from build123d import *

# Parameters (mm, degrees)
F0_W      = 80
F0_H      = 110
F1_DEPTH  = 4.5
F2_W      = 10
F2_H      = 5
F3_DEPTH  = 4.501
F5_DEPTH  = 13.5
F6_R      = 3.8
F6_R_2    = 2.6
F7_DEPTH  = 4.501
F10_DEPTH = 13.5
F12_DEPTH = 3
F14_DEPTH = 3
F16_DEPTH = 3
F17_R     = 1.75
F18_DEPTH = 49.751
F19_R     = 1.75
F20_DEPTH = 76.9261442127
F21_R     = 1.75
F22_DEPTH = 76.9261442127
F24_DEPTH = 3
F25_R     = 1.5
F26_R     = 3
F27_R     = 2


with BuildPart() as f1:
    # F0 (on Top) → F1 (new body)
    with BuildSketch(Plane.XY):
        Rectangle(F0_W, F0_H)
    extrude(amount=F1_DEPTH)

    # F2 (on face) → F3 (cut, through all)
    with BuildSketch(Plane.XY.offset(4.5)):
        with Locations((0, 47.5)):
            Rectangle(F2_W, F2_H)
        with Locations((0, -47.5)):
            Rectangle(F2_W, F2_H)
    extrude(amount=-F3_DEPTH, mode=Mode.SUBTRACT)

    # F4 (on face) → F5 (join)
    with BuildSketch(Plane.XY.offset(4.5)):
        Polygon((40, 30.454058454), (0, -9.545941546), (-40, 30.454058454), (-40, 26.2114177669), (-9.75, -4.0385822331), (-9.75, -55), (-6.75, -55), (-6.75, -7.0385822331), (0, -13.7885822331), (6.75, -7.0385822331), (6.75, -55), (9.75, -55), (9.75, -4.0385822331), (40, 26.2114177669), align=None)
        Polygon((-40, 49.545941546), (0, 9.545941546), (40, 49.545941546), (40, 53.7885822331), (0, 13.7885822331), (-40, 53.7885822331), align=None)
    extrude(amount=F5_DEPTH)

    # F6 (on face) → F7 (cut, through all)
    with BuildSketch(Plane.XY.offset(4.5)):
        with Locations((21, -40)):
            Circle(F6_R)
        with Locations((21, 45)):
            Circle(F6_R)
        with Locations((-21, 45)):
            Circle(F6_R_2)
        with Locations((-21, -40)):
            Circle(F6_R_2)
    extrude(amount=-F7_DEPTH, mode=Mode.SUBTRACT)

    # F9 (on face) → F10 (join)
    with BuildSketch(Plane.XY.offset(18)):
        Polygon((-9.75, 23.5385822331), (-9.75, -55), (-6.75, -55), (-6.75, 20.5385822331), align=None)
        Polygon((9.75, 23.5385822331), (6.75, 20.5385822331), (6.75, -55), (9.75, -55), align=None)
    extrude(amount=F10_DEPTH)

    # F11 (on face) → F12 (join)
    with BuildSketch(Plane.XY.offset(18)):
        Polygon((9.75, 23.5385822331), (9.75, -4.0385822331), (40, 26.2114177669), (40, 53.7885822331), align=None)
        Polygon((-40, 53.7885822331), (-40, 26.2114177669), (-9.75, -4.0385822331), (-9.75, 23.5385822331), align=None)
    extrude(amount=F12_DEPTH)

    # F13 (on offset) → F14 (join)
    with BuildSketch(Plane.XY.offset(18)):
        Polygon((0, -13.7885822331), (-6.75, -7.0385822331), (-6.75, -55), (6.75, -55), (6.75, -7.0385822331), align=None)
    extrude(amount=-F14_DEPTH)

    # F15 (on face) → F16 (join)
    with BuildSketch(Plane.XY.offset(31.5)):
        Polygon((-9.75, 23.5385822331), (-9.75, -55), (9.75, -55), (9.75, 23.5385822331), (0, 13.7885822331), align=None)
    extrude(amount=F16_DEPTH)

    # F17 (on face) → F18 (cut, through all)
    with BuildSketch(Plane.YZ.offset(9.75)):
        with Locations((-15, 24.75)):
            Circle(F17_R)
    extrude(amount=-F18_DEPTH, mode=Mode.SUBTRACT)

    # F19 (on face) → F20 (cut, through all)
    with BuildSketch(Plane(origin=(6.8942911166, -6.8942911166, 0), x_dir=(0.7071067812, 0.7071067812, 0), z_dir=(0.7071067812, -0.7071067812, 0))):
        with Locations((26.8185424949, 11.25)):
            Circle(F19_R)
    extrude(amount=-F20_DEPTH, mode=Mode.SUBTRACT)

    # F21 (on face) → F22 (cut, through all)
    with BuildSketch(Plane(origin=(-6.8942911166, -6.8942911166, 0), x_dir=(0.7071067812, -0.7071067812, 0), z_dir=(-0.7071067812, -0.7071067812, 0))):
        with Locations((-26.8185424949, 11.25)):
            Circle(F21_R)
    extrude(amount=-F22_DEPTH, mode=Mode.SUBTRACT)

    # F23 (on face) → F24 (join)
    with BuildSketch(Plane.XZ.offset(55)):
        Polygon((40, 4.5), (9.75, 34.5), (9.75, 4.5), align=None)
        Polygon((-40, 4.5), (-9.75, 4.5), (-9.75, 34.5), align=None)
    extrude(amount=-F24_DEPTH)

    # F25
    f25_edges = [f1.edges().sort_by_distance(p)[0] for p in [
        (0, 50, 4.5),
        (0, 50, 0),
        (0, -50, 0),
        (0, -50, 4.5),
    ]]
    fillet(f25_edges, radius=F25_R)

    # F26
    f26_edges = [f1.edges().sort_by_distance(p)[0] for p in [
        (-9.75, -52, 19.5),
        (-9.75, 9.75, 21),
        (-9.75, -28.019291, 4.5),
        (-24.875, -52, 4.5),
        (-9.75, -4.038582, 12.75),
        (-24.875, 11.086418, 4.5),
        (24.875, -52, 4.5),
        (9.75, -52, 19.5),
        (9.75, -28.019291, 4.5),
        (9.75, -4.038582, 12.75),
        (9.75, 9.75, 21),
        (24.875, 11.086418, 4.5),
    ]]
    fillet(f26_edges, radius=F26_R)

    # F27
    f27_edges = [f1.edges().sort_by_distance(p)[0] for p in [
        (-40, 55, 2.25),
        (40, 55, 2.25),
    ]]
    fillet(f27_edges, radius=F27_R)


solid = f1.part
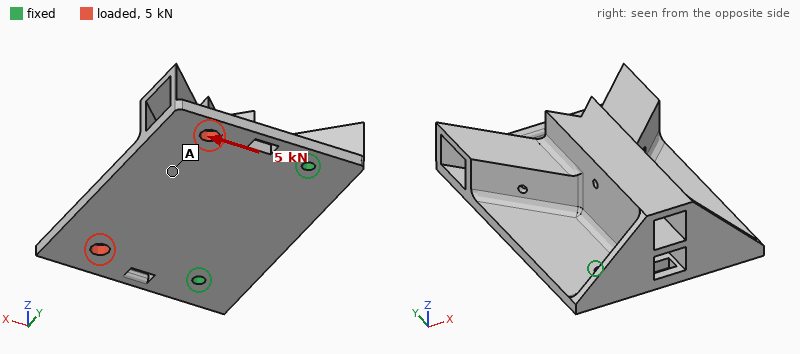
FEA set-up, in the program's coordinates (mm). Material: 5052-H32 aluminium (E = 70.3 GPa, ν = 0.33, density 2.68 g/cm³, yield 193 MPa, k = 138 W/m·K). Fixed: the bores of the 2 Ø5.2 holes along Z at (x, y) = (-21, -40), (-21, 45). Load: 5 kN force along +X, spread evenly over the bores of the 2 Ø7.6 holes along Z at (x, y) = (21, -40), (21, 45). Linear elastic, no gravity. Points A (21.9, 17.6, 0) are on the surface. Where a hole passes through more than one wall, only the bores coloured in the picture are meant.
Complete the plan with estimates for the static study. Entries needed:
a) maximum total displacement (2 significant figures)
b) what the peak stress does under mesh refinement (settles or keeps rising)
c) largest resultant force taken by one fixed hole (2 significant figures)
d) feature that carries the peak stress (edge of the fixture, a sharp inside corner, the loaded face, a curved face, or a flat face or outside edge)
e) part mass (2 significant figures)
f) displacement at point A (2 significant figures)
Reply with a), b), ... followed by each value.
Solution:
a) 23 µm
b) keeps rising
c) 2.5 kN
d) edge of the fixture
e) 190 g
f) 9.6 µm
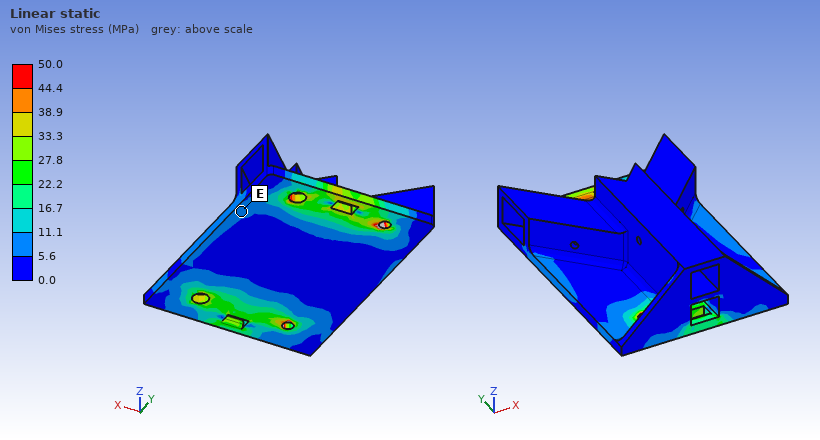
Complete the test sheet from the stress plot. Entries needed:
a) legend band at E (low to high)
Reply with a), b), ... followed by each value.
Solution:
a) 5.6 to 11.1 MPa
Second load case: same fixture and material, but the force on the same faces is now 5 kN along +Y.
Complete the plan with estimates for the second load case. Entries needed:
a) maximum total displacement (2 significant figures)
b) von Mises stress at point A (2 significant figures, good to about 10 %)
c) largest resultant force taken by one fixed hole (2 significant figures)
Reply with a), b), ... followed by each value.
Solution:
a) 46 µm
b) 15 MPa
c) 3.5 kN
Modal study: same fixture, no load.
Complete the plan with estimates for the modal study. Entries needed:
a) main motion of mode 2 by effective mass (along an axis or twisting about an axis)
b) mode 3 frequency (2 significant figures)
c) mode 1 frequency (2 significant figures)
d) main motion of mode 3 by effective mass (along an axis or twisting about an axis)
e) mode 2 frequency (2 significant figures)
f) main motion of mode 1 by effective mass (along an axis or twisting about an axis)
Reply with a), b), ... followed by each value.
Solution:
a) twisting about X
b) 4600 Hz
c) 880 Hz
d) along Z
e) 3300 Hz
f) along Z
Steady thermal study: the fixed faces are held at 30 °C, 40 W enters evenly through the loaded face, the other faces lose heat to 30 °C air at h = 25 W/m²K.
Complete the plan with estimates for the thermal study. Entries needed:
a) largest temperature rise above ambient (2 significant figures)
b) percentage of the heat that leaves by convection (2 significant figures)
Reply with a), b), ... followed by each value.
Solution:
a) 32 K
b) 32 %
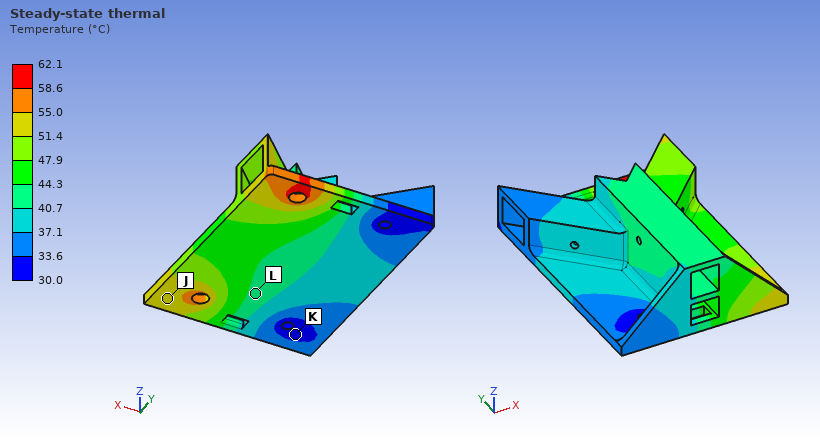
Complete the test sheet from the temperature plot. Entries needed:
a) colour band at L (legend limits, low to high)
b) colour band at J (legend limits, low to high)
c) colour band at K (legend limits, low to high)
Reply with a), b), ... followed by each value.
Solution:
a) 40.7 to 44.3 °C
b) 51.4 to 55.0 °C
c) 30.0 to 33.6 °C
